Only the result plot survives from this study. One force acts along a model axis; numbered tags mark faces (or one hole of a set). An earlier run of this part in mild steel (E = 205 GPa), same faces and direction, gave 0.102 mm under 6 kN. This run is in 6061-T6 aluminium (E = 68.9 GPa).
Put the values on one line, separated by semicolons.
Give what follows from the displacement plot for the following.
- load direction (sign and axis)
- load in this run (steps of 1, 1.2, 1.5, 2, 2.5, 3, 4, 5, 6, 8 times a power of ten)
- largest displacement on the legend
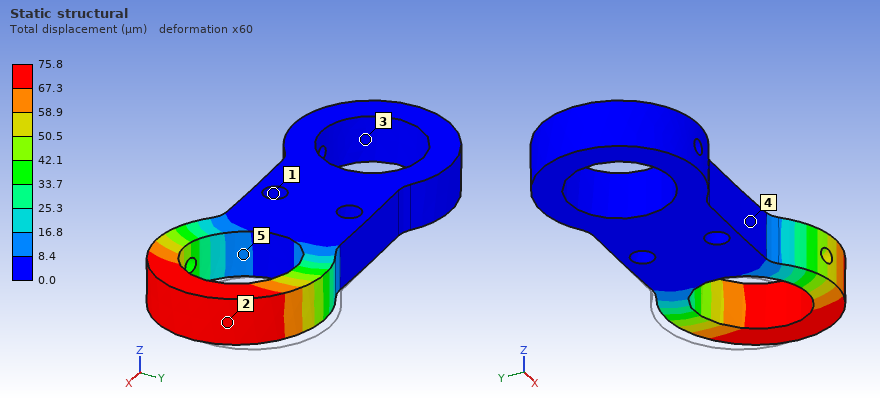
-Y; 1.5 kN; 75.8 µm
